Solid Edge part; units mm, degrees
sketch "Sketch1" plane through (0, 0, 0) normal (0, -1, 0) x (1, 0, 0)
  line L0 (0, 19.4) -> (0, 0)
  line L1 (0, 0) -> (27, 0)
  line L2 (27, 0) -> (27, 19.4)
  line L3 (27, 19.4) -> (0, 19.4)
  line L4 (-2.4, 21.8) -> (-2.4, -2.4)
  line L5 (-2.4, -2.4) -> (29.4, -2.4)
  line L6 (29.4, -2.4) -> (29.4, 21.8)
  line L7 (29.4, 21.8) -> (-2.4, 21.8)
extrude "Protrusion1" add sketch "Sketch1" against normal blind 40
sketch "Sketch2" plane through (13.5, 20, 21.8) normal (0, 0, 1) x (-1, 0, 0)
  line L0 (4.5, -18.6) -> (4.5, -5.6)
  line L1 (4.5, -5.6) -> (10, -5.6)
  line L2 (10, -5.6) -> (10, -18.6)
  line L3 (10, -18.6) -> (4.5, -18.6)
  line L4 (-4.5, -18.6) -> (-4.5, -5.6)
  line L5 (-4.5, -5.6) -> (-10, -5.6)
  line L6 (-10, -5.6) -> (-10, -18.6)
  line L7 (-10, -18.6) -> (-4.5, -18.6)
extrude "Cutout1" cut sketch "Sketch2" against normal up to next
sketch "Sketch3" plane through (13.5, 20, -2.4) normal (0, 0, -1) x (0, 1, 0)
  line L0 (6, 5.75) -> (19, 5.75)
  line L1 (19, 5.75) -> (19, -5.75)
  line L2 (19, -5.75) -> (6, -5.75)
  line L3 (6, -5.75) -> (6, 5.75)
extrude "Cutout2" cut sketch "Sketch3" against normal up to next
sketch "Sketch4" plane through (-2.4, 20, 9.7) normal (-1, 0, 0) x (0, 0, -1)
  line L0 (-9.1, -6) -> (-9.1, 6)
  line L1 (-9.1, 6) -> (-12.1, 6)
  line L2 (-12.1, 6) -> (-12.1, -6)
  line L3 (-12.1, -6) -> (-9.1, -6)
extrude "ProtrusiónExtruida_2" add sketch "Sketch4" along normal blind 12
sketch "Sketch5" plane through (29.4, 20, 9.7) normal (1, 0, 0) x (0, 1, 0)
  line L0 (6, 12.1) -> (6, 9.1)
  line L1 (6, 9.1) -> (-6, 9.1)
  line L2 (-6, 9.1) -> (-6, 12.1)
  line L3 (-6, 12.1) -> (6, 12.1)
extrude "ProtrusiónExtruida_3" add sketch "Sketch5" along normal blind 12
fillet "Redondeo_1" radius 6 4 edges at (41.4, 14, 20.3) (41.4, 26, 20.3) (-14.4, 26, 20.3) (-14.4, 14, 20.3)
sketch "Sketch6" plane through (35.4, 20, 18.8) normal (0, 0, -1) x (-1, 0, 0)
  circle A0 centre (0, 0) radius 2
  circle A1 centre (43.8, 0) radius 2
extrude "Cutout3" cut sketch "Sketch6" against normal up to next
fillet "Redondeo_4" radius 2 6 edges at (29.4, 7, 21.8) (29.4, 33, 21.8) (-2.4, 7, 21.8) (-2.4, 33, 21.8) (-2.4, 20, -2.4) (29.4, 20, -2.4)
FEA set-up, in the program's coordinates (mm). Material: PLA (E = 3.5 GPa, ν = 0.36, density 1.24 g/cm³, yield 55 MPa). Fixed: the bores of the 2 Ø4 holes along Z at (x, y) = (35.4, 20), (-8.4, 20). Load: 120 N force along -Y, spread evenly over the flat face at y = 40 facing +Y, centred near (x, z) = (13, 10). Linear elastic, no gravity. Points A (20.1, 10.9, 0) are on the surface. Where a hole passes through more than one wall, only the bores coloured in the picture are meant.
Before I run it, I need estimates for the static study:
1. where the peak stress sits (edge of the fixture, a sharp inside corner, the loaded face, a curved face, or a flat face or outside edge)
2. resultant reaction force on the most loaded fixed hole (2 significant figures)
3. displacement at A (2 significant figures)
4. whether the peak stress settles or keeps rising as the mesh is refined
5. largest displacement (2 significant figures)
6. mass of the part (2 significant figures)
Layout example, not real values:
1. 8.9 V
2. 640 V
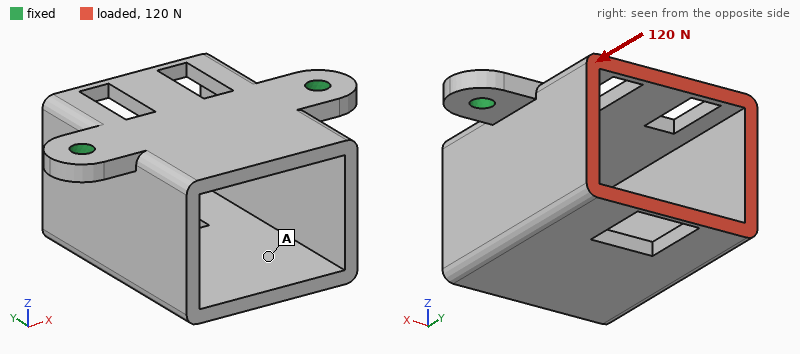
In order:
1. edge of the fixture
2. 60 N
3. 0.52 mm
4. keeps rising
5. 0.78 mm
6. 12 g
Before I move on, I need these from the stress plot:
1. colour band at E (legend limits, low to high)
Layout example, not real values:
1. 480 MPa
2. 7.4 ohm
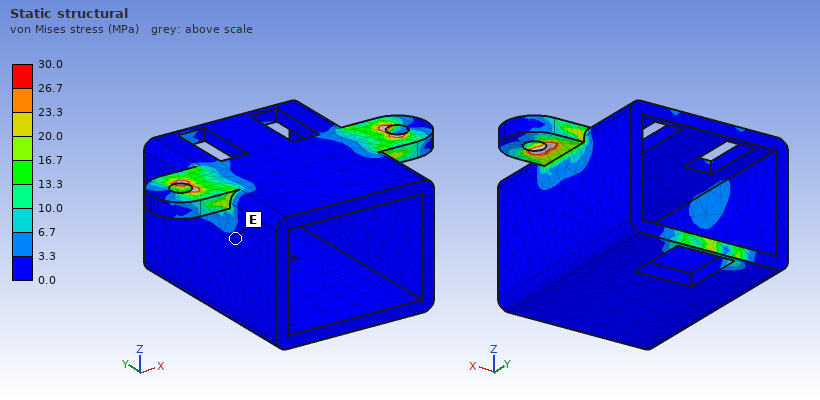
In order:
1. 0.0 to 3.3 MPa
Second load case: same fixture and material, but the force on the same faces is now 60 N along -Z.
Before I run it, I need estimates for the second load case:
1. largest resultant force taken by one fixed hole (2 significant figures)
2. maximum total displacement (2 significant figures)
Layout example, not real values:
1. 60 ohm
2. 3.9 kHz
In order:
1. 30 N
2. 0.74 mm
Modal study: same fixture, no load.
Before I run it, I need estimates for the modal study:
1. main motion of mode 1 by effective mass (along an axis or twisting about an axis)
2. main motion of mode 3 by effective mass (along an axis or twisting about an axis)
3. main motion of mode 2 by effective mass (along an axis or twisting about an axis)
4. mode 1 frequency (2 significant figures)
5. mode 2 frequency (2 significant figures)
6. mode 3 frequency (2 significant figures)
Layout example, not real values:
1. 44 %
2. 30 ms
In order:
1. along Y
2. twisting about Z
3. along X
4. 620 Hz
5. 1000 Hz
6. 1500 Hz
